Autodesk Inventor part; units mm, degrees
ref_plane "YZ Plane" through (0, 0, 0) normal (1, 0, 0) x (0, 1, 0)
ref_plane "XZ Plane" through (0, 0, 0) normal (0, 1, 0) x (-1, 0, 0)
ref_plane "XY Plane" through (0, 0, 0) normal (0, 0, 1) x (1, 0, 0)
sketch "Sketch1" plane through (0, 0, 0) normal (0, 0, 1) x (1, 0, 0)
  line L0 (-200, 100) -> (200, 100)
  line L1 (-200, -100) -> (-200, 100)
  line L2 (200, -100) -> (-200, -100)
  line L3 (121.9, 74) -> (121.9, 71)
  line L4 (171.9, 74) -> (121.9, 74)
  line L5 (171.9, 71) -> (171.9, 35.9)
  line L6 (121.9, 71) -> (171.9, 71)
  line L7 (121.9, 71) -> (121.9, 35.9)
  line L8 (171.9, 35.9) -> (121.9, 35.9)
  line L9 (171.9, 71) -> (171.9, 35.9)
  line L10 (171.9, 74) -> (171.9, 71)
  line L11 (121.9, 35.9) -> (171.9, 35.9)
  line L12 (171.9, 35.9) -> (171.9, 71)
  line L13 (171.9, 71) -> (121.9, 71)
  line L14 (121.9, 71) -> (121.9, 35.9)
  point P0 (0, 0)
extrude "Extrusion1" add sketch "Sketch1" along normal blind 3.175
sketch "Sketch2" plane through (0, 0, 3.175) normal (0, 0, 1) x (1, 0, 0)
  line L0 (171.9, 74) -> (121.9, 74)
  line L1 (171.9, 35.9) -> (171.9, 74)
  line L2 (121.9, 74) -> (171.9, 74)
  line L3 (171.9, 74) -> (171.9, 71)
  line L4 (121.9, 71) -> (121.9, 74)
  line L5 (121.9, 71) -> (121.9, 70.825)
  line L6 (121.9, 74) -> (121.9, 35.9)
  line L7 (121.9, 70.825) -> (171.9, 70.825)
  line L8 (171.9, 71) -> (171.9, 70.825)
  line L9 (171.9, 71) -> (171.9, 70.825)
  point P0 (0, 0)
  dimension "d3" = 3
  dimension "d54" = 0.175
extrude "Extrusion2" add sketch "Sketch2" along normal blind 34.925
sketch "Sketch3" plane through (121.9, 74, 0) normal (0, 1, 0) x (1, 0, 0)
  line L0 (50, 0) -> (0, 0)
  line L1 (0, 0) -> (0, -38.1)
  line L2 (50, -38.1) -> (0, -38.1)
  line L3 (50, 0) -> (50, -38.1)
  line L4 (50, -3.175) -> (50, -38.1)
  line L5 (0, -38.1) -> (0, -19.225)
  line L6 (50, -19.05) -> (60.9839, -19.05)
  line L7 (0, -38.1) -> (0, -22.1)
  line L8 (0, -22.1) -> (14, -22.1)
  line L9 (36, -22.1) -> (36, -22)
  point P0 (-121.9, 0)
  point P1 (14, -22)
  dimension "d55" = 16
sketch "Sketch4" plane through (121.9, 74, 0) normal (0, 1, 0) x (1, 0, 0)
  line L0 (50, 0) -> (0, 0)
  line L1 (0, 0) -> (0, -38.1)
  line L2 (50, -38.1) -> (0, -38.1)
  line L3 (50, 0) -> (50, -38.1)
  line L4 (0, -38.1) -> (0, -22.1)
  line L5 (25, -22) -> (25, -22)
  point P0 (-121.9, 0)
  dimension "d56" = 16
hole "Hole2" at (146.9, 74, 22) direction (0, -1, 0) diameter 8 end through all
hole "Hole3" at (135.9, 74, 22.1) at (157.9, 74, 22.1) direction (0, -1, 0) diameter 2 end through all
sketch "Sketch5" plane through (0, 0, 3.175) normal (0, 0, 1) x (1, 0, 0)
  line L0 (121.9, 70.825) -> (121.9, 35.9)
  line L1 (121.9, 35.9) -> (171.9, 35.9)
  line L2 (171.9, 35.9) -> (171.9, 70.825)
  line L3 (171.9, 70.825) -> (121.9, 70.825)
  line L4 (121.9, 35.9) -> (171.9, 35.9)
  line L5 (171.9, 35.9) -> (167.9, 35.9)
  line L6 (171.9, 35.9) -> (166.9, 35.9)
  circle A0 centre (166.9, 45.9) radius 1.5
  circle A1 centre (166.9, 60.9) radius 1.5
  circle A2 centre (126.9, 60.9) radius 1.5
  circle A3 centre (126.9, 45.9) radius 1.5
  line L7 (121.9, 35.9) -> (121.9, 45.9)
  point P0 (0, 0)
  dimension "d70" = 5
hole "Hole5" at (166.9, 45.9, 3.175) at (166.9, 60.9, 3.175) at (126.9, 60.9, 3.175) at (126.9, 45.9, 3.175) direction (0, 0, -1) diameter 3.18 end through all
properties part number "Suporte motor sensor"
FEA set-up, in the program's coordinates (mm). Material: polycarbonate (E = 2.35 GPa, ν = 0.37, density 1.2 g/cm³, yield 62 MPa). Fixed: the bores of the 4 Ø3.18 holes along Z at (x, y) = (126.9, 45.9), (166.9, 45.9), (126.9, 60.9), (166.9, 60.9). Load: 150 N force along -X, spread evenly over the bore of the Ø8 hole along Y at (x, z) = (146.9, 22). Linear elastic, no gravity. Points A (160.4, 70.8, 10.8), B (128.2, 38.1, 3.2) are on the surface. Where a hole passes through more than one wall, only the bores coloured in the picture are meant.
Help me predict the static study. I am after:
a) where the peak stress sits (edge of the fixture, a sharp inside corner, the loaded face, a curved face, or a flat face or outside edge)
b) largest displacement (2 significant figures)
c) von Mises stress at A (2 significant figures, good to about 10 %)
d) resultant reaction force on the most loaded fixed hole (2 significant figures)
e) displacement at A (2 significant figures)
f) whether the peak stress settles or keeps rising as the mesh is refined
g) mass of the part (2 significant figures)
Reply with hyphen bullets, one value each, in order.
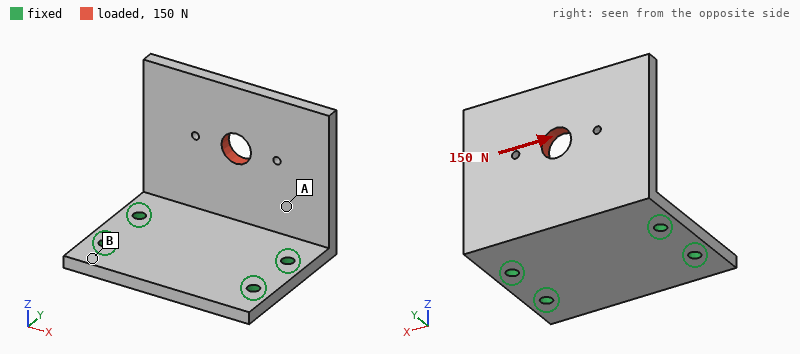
- edge of the fixture
- 0.71 mm
- 5.5 MPa
- 110 N
- 0.23 mm
- keeps rising
- 14 g
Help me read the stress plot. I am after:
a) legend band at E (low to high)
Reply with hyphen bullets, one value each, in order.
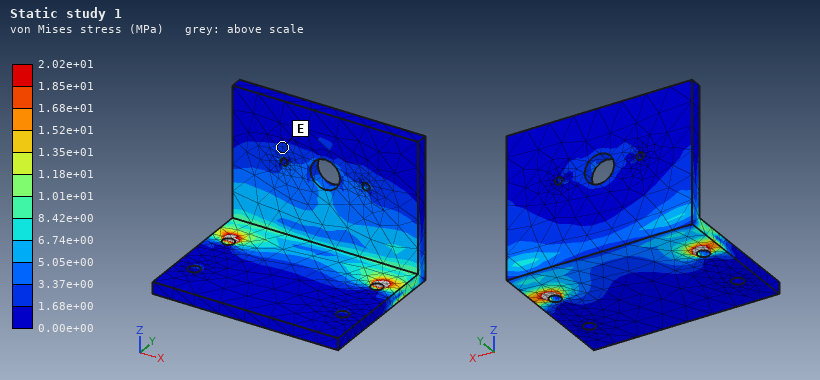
- 1.68e+00 to 3.37e+00 MPa
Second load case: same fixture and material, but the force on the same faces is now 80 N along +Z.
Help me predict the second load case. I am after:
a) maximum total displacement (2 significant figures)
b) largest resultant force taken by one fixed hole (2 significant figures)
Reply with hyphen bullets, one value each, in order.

- 0.73 mm
- 50 N
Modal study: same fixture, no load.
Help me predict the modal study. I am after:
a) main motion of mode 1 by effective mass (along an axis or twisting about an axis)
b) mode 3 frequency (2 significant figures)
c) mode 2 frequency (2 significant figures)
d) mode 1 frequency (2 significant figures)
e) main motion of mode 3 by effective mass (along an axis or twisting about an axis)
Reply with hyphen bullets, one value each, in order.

- along Y
- 1300 Hz
- 820 Hz
- 370 Hz
- along X
